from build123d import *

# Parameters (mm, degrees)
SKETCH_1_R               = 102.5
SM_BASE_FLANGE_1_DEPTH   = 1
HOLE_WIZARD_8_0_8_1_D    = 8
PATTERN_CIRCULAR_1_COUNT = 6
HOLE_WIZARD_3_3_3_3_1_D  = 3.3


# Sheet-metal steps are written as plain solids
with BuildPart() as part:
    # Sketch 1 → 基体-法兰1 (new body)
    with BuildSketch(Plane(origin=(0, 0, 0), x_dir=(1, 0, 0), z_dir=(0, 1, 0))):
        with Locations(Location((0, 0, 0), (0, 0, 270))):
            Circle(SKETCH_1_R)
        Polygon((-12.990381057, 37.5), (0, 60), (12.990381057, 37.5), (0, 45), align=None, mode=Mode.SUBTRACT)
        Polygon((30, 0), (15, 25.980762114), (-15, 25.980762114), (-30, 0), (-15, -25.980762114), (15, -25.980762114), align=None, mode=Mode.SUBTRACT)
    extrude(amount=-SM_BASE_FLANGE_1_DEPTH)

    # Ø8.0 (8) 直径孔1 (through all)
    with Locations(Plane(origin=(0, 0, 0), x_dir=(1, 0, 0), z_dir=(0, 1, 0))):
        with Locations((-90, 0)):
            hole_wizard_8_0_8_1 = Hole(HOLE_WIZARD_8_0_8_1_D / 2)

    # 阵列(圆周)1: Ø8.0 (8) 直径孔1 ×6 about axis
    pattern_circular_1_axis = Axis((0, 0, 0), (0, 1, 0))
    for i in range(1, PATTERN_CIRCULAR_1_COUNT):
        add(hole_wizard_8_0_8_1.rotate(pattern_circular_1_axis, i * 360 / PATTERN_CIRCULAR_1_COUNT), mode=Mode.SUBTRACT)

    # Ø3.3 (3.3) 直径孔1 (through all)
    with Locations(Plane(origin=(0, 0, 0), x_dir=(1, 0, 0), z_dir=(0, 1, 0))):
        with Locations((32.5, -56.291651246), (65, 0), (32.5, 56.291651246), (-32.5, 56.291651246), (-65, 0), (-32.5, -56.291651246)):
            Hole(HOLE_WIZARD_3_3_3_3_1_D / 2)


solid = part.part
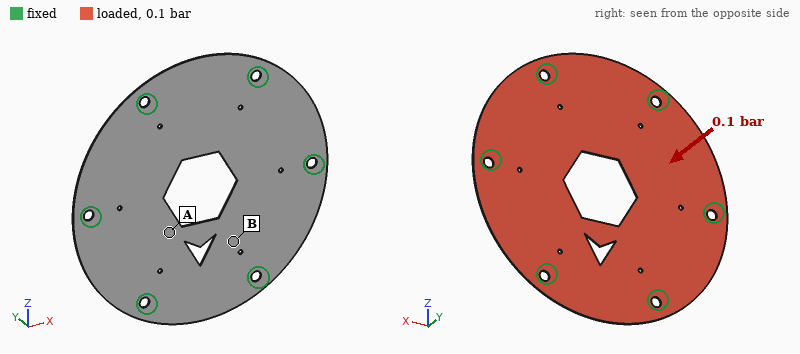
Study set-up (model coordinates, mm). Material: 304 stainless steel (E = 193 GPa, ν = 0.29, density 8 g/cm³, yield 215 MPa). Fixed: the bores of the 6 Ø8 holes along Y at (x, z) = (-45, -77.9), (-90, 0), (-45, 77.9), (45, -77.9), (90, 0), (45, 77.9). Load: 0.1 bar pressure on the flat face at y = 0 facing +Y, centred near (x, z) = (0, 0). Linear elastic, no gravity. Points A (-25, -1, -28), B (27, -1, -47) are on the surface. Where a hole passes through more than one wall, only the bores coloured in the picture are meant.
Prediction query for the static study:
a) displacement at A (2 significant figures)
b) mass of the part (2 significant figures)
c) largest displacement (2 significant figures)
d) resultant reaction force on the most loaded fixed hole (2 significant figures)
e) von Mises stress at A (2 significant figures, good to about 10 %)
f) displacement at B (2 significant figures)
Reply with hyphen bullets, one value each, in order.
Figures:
- 0.50 mm
- 240 g
- 0.63 mm
- 50 N
- 26 MPa
- 0.31 mm
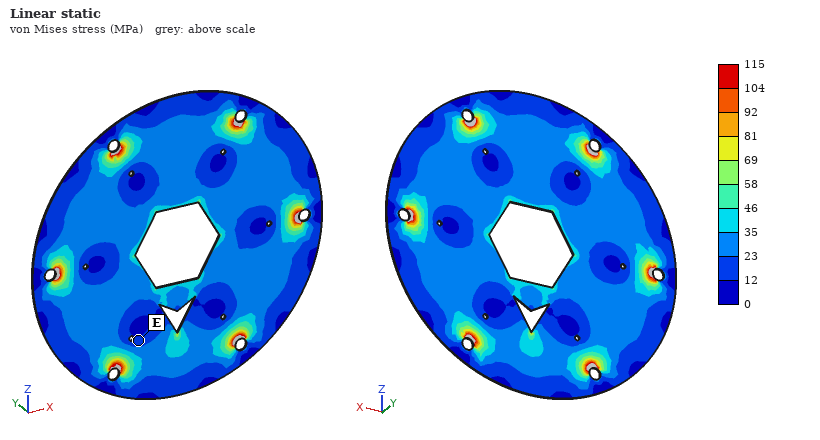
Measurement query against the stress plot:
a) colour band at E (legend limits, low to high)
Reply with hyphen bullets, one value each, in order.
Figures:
- 12 to 23 MPa
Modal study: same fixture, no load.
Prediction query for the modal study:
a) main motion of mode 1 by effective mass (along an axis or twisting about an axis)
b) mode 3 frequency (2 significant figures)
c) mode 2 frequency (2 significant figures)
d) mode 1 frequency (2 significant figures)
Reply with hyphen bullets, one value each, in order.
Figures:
- along Y
- 490 Hz
- 490 Hz
- 290 Hz
